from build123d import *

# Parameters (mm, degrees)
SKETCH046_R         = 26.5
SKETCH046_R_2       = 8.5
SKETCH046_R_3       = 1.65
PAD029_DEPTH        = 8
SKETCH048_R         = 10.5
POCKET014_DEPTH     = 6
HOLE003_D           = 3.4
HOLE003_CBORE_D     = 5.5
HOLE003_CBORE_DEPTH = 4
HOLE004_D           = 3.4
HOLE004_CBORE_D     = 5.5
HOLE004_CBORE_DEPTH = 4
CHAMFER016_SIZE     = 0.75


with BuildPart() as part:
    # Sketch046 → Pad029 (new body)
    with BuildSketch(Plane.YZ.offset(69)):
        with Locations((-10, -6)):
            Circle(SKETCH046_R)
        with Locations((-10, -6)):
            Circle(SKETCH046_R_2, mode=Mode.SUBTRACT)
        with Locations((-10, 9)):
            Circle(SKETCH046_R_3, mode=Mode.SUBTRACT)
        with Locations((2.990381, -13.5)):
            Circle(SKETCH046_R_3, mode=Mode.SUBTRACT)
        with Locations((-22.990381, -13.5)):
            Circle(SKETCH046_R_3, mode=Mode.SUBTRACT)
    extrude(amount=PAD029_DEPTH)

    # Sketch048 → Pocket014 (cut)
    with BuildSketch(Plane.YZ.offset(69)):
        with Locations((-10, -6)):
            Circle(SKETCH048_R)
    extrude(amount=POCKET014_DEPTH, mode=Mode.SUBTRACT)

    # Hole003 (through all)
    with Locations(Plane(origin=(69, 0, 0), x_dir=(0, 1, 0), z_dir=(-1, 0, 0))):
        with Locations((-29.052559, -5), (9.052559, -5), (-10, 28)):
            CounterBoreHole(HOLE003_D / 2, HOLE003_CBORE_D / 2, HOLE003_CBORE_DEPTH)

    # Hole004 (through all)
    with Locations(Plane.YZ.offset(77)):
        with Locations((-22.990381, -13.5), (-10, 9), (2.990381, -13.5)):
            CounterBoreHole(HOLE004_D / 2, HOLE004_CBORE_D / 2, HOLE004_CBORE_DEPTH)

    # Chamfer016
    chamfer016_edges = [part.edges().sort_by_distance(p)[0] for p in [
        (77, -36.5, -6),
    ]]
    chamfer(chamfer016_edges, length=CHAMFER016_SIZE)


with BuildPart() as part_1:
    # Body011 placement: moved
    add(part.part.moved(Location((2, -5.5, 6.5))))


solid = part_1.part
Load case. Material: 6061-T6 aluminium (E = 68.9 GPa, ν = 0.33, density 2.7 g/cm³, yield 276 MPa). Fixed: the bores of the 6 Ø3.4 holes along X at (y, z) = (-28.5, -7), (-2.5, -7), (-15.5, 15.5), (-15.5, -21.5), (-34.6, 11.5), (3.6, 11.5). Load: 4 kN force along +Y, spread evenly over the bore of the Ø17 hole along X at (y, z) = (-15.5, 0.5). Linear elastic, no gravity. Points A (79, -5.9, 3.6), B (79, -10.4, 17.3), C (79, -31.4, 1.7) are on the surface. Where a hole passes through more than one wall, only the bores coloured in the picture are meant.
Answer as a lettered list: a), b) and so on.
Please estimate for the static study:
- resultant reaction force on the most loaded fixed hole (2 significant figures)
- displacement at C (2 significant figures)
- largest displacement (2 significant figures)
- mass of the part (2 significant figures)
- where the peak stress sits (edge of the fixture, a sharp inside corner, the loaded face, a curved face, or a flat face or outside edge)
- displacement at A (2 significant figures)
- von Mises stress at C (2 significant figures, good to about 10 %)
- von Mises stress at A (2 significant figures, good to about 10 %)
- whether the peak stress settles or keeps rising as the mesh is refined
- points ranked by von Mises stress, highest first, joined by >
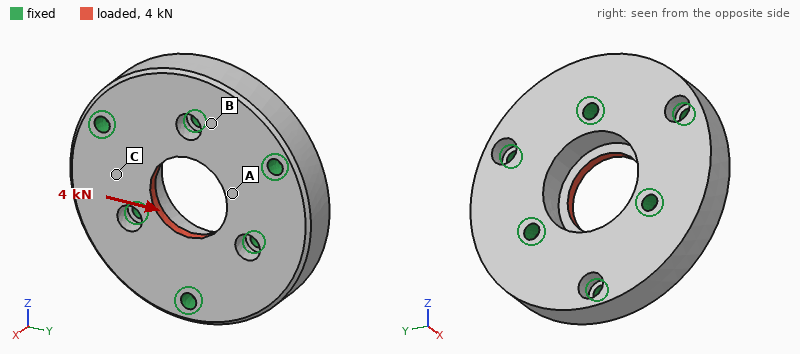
a) 760 N
b) 3.2 µm
c) 9.2 µm
d) 39 g
e) edge of the fixture
f) 5.7 µm
g) 17 MPa
h) 40 MPa
i) keeps rising
j) A > C > B
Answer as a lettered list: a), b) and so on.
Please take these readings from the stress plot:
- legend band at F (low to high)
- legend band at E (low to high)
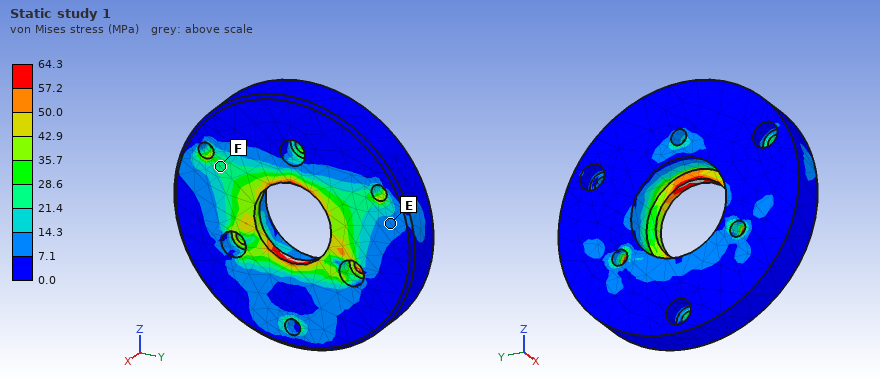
a) 21.4 to 28.6 MPa
b) 7.1 to 14.3 MPa
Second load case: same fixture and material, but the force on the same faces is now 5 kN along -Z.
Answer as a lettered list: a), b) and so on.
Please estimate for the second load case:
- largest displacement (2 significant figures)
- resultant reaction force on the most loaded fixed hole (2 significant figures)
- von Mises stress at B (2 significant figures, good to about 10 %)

a) 13 µm
b) 1.0 kN
c) 16 MPa
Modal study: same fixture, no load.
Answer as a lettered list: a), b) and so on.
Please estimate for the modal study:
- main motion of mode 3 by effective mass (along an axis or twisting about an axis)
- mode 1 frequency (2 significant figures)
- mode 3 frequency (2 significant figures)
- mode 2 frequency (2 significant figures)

a) along X
b) 25 kHz
c) 27 kHz
d) 25 kHz
